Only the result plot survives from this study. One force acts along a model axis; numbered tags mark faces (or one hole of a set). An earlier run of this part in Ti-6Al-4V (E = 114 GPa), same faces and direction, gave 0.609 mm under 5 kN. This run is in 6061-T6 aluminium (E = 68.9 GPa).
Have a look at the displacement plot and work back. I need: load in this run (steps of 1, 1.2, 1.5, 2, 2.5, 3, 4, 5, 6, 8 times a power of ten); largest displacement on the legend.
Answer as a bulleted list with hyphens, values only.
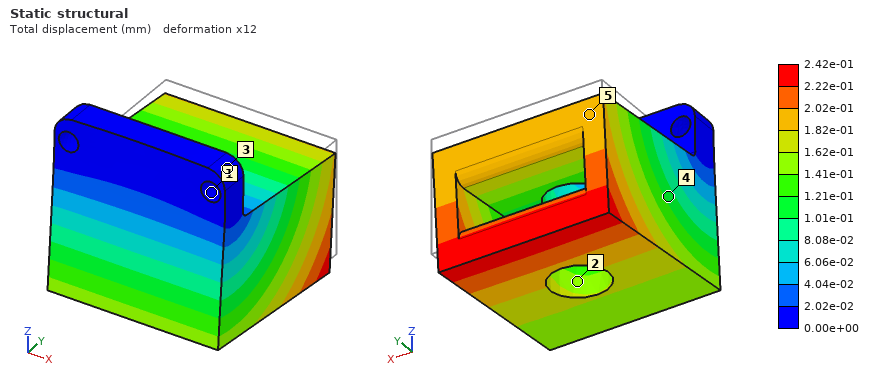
- 1.2 kN
- 2.42e-01 mm
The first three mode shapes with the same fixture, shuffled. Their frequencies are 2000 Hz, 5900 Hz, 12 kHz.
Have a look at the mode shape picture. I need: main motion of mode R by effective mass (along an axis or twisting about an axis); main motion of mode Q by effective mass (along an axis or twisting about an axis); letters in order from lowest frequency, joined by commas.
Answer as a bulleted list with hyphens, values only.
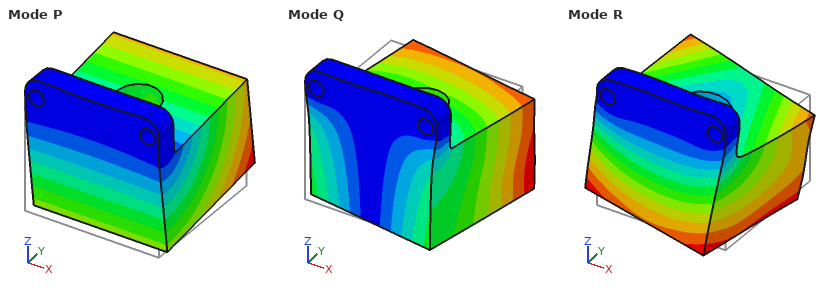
- along X
- along X
- P, Q, R
